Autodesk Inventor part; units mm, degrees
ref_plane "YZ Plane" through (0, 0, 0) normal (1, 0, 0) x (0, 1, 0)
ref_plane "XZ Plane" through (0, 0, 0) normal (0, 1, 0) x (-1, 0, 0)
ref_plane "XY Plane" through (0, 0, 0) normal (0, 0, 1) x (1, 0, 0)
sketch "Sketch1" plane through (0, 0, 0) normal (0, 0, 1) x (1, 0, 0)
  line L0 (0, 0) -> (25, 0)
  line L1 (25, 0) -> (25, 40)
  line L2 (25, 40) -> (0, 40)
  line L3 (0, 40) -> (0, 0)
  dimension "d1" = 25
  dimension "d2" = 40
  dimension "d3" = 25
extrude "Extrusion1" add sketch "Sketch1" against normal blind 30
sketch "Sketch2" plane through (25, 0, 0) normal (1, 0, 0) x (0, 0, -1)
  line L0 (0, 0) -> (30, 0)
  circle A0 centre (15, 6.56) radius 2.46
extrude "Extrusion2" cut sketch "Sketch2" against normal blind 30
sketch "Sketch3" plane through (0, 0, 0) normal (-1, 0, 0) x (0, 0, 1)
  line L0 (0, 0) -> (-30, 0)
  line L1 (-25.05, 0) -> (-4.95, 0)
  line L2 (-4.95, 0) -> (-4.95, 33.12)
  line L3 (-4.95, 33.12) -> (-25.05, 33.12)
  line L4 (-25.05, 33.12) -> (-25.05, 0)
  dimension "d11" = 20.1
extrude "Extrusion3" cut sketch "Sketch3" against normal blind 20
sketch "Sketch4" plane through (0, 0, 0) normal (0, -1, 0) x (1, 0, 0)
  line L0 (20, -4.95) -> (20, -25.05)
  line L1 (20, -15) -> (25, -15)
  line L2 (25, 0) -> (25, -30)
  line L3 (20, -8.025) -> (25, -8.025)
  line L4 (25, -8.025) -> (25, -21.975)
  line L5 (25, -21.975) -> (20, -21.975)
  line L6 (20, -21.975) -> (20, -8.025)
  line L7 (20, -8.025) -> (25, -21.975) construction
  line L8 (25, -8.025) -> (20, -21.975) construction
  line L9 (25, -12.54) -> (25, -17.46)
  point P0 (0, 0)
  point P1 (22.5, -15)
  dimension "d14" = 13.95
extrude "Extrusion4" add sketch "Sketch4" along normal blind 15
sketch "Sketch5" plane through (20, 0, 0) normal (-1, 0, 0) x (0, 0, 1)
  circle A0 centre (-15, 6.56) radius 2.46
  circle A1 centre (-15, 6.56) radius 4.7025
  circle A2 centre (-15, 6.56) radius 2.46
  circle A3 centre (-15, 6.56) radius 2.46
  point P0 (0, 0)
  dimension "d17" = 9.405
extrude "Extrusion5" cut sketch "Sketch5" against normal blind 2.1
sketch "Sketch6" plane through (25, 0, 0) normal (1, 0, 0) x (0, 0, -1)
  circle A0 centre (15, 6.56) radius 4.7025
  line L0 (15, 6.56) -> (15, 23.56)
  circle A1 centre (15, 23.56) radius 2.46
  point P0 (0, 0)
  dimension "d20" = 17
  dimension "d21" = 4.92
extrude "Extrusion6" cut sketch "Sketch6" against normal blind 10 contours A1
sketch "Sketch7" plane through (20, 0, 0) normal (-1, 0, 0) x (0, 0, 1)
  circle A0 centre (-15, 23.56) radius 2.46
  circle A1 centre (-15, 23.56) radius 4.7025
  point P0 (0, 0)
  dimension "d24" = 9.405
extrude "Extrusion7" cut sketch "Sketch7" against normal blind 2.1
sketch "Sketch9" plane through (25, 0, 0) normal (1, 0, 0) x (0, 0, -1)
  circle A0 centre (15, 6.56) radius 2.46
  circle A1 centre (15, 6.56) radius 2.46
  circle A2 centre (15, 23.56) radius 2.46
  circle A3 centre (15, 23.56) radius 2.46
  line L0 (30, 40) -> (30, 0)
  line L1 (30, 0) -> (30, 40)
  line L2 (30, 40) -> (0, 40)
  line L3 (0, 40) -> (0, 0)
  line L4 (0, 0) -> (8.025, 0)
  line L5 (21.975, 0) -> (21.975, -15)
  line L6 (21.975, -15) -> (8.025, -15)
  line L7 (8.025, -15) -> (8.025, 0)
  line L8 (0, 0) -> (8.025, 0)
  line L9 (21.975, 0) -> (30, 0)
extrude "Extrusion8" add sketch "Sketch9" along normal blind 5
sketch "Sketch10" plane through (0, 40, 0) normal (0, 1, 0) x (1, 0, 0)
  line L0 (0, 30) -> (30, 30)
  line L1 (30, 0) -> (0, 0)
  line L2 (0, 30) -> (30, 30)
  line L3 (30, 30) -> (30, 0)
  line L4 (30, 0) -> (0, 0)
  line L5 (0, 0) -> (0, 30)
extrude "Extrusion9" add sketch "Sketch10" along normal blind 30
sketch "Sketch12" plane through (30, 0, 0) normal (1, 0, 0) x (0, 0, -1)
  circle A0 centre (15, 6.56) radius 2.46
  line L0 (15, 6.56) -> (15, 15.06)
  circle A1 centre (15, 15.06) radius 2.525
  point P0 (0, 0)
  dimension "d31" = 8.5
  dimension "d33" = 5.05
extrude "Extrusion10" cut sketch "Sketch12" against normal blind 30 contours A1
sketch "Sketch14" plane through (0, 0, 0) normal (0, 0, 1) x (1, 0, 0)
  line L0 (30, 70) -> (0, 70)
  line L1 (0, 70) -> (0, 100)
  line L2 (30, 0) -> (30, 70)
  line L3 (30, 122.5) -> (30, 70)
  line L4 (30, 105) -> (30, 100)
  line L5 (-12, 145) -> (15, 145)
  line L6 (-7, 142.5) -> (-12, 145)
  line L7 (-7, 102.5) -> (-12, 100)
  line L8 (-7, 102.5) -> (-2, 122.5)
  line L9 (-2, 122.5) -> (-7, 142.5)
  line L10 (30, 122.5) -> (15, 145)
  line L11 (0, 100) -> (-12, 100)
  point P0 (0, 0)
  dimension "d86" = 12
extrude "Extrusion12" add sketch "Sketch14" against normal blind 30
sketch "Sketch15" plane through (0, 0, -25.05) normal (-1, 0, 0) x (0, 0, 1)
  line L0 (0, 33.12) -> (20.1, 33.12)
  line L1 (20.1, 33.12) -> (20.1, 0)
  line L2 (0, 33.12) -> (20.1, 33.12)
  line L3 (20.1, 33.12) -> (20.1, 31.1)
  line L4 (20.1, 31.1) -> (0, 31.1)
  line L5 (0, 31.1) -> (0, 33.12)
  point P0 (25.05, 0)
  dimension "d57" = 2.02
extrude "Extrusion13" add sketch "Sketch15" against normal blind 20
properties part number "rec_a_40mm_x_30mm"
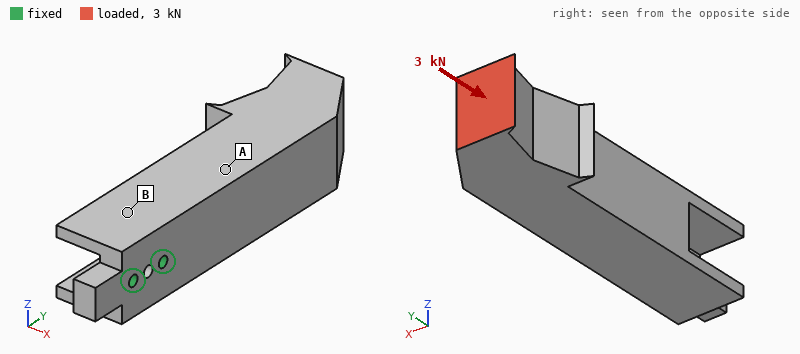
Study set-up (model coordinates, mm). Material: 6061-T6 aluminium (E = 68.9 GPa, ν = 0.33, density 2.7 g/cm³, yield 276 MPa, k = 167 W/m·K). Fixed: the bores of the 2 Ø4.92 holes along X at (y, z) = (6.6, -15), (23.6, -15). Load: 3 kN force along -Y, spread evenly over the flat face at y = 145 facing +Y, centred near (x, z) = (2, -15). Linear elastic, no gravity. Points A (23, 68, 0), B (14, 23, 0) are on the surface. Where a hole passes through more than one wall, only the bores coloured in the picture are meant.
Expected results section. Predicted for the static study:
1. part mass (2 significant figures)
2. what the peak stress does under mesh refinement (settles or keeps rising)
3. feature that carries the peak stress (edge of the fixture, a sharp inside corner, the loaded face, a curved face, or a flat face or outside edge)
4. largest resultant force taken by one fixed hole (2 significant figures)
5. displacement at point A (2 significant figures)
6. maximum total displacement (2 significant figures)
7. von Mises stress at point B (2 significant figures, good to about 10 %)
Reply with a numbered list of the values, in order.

1. 330 g
2. keeps rising
3. edge of the fixture
4. 3.4 kN
5. 0.076 mm
6. 0.27 mm
7. 21 MPa
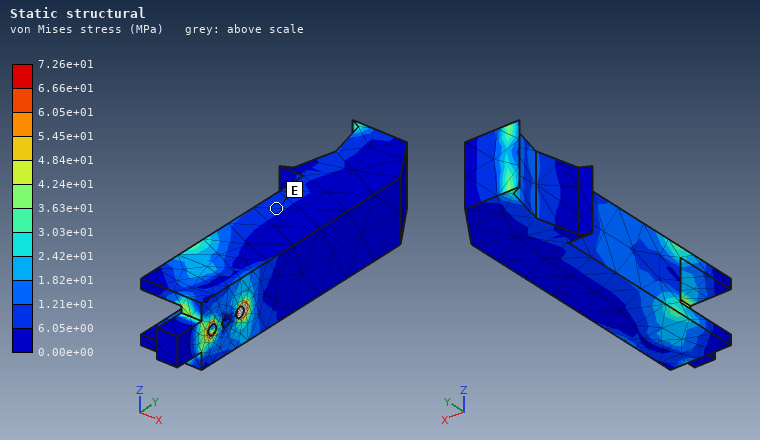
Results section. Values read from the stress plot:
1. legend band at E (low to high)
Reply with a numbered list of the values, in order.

1. 6.05e+00 to 1.21e+01 MPa
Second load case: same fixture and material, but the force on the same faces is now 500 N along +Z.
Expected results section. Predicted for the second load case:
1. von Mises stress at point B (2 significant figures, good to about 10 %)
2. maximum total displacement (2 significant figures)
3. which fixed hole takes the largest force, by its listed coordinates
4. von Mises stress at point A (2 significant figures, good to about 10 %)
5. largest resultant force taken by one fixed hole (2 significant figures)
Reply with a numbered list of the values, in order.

1. 18 MPa
2. 0.18 mm
3. (23.6, -15)
4. 8.8 MPa
5. 3.1 kN
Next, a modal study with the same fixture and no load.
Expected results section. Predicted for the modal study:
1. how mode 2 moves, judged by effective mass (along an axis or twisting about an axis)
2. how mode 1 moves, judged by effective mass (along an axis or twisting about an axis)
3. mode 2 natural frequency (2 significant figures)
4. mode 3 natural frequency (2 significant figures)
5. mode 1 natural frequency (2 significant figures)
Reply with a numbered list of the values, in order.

1. along Z
2. along X
3. 910 Hz
4. 2900 Hz
5. 780 Hz
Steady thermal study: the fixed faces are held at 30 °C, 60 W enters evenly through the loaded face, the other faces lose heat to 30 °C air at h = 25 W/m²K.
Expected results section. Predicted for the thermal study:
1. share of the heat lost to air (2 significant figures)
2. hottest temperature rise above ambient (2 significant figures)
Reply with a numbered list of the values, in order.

1. 20 %
2. 62 K
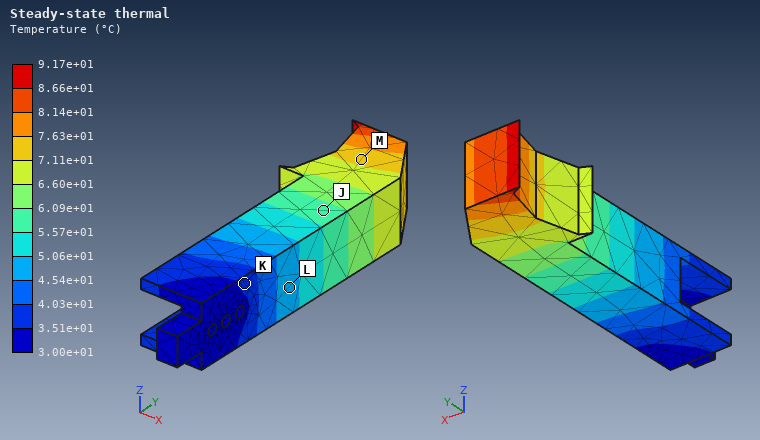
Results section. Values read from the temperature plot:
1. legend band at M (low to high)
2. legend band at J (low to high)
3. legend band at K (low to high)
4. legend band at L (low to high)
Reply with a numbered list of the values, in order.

1. 7.11e+01 to 7.63e+01 °C
2. 5.57e+01 to 6.09e+01 °C
3. 3.51e+01 to 4.03e+01 °C
4. 4.54e+01 to 5.06e+01 °C
